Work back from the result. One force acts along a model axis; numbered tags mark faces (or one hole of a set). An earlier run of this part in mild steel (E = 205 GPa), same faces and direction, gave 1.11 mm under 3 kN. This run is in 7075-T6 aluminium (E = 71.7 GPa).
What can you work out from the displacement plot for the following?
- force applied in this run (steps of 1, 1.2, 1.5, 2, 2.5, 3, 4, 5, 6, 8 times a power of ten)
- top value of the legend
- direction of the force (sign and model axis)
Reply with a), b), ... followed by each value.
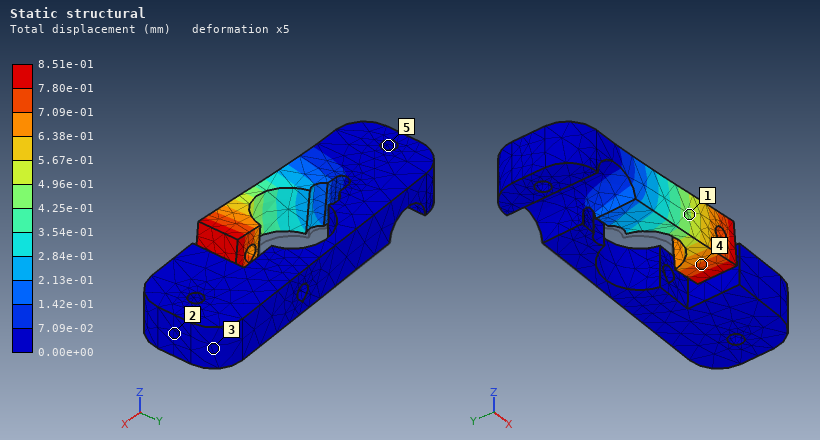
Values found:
a) 800 N
b) 8.51e-01 mm
c) +Z
